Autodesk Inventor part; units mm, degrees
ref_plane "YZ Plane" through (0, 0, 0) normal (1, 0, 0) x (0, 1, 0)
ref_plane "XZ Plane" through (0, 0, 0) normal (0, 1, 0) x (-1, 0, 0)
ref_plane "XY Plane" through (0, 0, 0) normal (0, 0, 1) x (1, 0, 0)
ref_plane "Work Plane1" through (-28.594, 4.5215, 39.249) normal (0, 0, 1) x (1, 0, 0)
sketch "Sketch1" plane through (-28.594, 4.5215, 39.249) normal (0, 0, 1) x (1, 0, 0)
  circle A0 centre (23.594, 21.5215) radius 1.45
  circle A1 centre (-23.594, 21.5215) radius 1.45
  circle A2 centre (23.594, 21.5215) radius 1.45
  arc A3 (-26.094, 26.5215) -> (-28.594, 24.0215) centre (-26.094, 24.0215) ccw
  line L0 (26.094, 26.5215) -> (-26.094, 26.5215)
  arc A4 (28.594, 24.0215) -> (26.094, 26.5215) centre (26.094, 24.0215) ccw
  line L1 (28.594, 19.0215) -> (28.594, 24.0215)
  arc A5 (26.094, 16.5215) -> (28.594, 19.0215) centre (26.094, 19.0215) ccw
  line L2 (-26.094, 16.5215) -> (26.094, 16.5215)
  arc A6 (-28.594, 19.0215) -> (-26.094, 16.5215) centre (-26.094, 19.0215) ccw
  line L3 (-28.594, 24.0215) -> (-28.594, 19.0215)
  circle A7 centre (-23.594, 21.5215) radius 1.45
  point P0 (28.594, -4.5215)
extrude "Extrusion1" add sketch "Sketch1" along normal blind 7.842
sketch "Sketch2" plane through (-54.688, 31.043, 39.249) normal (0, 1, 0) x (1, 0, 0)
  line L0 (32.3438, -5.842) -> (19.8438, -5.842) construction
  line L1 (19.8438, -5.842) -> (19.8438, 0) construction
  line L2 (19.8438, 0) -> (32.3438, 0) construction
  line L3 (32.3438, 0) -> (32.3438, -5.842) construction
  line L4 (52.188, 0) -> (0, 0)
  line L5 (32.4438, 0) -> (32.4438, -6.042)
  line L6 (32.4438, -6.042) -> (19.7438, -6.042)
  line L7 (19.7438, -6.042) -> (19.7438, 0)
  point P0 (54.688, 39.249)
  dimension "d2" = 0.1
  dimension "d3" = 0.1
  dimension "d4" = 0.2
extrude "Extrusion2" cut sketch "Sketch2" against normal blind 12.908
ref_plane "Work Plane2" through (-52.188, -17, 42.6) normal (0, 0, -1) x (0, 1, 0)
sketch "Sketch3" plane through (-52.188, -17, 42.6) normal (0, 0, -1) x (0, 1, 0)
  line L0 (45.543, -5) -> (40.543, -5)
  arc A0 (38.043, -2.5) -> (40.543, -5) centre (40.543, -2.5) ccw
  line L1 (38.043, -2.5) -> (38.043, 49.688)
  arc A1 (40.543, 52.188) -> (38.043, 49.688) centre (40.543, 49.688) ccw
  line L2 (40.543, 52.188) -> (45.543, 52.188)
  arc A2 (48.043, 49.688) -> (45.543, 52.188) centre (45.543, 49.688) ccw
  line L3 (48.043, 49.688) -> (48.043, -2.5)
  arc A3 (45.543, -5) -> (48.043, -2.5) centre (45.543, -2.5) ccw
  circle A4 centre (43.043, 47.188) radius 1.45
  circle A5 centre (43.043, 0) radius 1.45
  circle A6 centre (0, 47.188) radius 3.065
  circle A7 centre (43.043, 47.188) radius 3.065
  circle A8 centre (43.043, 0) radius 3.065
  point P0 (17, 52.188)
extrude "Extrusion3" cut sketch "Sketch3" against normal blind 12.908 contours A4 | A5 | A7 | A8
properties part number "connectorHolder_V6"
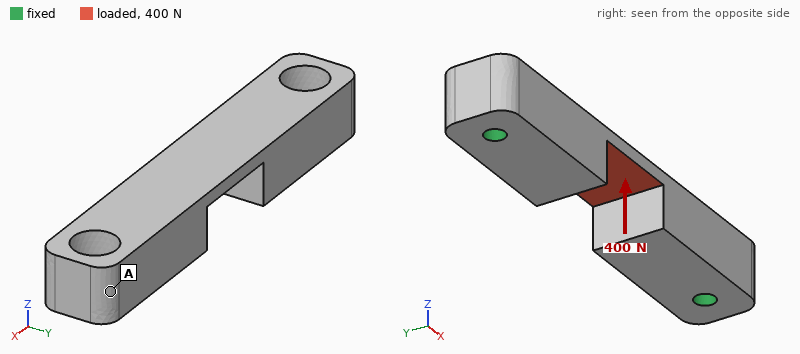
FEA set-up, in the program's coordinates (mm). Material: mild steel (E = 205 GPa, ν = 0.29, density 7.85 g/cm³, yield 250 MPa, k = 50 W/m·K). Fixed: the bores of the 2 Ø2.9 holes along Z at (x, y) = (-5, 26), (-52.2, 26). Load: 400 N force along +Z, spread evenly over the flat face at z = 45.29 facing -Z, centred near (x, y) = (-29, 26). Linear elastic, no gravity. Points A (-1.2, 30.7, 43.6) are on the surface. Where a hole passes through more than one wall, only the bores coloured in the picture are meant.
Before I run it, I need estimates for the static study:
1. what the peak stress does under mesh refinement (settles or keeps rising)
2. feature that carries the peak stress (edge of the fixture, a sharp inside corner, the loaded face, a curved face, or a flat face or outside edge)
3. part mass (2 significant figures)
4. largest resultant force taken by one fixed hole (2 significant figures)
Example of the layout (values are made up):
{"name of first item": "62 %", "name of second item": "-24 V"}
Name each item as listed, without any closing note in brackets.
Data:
{"what the peak stress does under mesh refinement": "keeps rising", "feature that carries the peak stress": "edge of the fixture", "part mass": "26 g", "largest resultant force taken by one fixed hole": "510 N"}
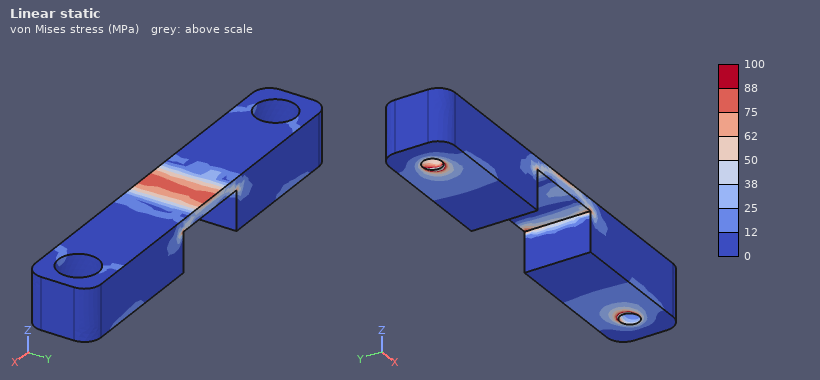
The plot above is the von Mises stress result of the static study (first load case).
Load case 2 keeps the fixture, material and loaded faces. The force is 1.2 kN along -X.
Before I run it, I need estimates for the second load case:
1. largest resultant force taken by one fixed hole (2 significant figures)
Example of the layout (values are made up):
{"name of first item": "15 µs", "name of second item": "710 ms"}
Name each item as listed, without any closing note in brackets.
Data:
{"largest resultant force taken by one fixed hole": "600 N"}
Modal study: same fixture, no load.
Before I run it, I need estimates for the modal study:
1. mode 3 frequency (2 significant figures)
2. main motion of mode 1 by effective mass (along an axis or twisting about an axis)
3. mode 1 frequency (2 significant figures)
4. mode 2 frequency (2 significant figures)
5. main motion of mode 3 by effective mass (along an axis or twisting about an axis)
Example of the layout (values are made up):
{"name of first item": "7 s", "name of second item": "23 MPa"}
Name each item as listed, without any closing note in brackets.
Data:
{"mode 3 frequency": "14 kHz", "main motion of mode 1 by effective mass": "along Y", "mode 1 frequency": "12 kHz", "mode 2 frequency": "13 kHz", "main motion of mode 3 by effective mass": "along Z"}
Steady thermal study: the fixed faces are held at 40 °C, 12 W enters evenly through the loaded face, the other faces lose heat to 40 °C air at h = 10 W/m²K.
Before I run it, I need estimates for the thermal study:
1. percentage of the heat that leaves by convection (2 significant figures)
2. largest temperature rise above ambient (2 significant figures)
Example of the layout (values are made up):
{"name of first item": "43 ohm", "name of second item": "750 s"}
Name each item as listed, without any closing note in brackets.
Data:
{"percentage of the heat that leaves by convection": "3.1 %", "largest temperature rise above ambient": "61 K"}
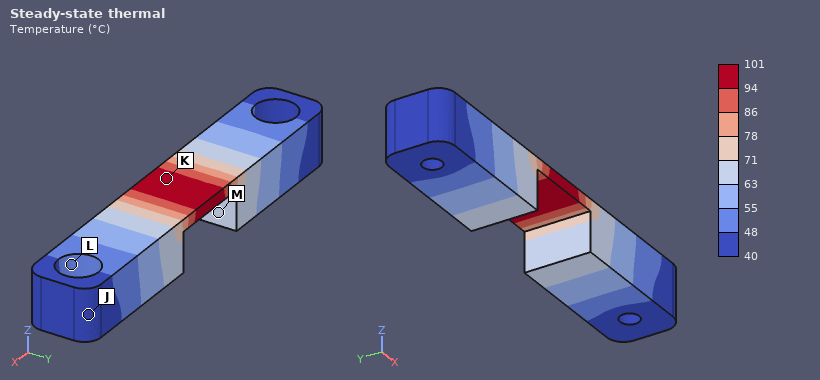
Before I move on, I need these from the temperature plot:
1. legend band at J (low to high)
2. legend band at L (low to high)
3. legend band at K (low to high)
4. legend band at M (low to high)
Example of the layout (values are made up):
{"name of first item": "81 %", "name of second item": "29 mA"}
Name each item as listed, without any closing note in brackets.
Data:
{"legend band at J": "40 to 48 °C", "legend band at L": "48 to 55 °C", "legend band at K": "94 to 101 °C", "legend band at M": "63 to 71 °C"}
